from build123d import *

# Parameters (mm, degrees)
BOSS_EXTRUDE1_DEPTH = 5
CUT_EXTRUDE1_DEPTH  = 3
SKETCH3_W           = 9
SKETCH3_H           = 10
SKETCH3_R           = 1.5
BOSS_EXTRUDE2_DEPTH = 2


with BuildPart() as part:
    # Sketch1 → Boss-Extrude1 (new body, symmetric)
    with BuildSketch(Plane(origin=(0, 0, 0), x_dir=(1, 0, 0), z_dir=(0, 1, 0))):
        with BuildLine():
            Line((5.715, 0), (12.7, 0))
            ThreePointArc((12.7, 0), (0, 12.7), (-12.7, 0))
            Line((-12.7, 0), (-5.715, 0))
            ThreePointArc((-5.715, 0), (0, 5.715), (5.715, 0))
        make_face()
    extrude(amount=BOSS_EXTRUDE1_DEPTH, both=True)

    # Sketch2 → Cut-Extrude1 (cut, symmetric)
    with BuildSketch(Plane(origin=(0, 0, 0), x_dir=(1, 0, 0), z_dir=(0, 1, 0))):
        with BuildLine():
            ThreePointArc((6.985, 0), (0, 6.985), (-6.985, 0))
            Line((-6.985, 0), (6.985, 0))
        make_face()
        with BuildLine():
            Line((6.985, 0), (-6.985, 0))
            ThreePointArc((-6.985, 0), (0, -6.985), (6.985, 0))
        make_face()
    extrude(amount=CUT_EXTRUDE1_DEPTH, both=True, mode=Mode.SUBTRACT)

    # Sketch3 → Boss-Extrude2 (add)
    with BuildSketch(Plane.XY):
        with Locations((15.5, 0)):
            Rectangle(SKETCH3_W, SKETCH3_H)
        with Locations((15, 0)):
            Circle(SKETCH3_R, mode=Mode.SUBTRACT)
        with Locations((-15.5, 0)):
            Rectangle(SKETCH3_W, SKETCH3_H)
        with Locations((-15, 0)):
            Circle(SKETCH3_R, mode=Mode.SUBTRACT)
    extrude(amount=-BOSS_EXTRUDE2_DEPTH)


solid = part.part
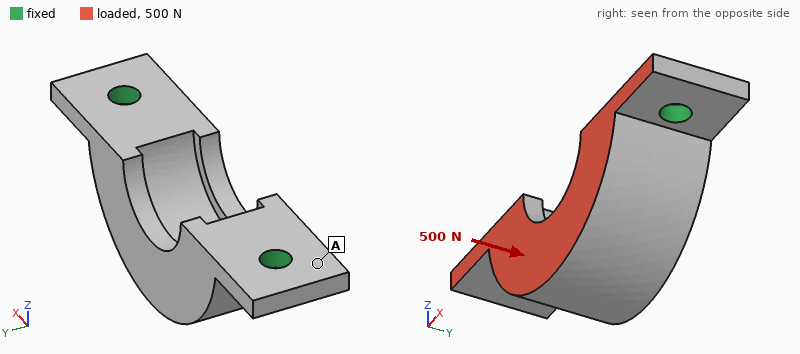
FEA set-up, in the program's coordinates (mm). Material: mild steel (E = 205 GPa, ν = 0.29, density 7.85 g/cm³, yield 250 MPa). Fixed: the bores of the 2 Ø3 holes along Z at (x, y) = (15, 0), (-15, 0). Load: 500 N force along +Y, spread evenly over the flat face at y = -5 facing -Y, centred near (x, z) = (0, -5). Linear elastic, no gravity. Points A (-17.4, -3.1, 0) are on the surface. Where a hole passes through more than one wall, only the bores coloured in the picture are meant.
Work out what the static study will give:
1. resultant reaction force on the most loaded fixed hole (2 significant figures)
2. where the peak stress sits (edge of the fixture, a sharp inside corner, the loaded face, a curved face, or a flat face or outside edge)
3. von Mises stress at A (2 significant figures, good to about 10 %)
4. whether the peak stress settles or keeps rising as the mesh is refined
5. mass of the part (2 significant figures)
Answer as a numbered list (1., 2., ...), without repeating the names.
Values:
1. 250 N
2. edge of the fixture
3. 34 MPa
4. keeps rising
5. 17 g
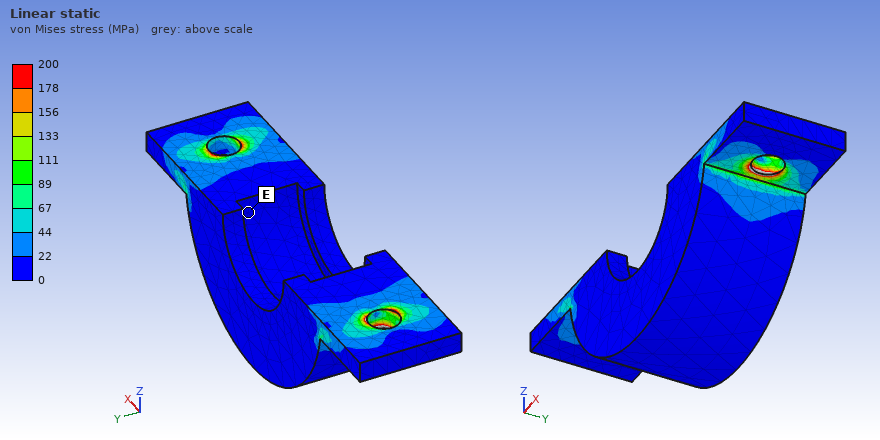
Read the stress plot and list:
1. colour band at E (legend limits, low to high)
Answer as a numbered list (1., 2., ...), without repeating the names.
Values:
1. 0 to 22 MPa
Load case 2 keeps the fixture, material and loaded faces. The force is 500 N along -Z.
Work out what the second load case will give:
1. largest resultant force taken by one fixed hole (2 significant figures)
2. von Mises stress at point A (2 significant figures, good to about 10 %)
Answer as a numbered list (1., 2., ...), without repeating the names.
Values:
1. 300 N
2. 35 MPa
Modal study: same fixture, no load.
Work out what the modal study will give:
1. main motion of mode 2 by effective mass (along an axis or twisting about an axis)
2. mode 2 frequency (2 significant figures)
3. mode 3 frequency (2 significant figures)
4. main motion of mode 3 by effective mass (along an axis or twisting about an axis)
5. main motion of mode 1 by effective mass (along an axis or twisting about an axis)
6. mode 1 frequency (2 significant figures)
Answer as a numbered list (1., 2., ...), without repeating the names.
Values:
1. along Z
2. 25 kHz
3. 35 kHz
4. along X
5. along Y
6. 8300 Hz
